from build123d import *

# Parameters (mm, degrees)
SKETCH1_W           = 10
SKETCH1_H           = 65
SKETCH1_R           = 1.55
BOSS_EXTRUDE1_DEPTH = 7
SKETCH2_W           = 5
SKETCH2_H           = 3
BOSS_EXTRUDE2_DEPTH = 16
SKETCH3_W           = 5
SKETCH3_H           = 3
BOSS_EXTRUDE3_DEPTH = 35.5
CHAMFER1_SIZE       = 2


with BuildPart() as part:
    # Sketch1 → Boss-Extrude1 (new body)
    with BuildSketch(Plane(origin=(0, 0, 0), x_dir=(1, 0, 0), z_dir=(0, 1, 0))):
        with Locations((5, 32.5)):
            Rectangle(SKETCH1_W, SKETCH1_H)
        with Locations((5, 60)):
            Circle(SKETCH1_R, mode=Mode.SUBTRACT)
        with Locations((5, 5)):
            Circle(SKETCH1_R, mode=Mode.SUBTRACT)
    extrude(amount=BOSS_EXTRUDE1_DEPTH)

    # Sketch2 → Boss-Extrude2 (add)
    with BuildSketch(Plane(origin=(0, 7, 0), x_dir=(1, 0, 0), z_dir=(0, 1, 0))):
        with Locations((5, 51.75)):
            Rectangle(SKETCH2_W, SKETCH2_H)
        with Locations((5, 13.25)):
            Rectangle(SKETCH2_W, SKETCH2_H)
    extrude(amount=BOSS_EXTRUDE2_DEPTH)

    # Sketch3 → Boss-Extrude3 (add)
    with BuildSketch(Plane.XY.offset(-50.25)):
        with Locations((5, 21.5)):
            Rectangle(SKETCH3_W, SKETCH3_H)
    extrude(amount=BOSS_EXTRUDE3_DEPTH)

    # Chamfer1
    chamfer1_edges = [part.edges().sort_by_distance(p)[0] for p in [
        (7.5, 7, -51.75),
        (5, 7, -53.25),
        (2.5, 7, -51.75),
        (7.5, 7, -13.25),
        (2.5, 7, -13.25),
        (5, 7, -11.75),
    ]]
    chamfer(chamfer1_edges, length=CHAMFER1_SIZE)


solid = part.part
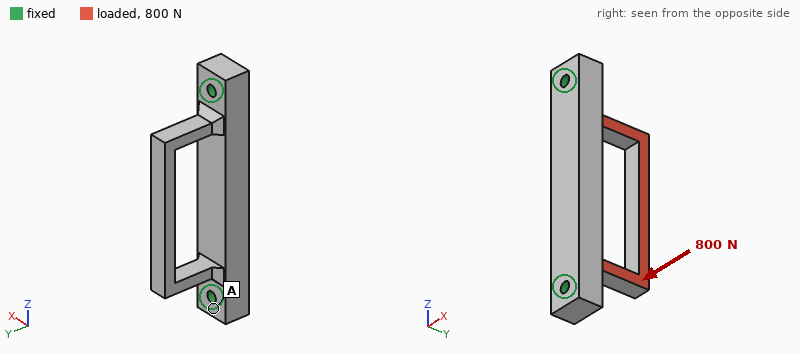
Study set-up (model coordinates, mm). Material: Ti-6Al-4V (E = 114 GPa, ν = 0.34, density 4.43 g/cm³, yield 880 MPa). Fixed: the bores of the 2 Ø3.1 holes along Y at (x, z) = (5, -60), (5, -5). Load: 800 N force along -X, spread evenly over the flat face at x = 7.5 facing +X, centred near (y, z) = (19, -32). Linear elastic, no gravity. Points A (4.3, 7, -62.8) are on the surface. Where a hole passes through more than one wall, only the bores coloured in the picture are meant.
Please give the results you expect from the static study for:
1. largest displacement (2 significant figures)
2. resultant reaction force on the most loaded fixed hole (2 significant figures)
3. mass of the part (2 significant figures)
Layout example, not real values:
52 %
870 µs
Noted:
0.20 mm
400 N
24 g
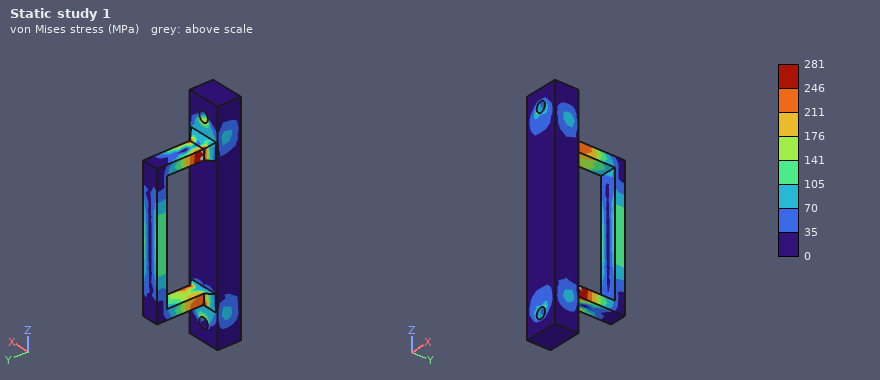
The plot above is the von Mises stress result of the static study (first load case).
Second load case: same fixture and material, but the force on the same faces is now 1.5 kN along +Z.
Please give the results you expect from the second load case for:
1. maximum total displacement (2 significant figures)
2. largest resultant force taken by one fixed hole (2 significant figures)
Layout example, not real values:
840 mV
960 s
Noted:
0.23 mm
830 N
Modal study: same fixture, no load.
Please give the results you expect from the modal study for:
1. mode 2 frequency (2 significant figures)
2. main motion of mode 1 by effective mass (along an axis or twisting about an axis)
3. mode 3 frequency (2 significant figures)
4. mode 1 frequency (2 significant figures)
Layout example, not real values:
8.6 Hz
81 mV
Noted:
6700 Hz
along X
8500 Hz
5700 Hz
